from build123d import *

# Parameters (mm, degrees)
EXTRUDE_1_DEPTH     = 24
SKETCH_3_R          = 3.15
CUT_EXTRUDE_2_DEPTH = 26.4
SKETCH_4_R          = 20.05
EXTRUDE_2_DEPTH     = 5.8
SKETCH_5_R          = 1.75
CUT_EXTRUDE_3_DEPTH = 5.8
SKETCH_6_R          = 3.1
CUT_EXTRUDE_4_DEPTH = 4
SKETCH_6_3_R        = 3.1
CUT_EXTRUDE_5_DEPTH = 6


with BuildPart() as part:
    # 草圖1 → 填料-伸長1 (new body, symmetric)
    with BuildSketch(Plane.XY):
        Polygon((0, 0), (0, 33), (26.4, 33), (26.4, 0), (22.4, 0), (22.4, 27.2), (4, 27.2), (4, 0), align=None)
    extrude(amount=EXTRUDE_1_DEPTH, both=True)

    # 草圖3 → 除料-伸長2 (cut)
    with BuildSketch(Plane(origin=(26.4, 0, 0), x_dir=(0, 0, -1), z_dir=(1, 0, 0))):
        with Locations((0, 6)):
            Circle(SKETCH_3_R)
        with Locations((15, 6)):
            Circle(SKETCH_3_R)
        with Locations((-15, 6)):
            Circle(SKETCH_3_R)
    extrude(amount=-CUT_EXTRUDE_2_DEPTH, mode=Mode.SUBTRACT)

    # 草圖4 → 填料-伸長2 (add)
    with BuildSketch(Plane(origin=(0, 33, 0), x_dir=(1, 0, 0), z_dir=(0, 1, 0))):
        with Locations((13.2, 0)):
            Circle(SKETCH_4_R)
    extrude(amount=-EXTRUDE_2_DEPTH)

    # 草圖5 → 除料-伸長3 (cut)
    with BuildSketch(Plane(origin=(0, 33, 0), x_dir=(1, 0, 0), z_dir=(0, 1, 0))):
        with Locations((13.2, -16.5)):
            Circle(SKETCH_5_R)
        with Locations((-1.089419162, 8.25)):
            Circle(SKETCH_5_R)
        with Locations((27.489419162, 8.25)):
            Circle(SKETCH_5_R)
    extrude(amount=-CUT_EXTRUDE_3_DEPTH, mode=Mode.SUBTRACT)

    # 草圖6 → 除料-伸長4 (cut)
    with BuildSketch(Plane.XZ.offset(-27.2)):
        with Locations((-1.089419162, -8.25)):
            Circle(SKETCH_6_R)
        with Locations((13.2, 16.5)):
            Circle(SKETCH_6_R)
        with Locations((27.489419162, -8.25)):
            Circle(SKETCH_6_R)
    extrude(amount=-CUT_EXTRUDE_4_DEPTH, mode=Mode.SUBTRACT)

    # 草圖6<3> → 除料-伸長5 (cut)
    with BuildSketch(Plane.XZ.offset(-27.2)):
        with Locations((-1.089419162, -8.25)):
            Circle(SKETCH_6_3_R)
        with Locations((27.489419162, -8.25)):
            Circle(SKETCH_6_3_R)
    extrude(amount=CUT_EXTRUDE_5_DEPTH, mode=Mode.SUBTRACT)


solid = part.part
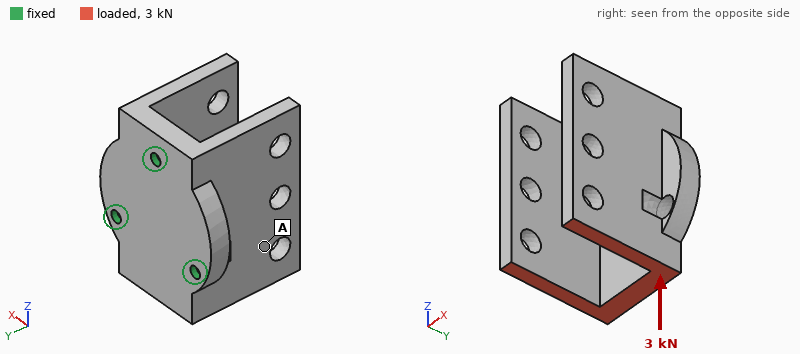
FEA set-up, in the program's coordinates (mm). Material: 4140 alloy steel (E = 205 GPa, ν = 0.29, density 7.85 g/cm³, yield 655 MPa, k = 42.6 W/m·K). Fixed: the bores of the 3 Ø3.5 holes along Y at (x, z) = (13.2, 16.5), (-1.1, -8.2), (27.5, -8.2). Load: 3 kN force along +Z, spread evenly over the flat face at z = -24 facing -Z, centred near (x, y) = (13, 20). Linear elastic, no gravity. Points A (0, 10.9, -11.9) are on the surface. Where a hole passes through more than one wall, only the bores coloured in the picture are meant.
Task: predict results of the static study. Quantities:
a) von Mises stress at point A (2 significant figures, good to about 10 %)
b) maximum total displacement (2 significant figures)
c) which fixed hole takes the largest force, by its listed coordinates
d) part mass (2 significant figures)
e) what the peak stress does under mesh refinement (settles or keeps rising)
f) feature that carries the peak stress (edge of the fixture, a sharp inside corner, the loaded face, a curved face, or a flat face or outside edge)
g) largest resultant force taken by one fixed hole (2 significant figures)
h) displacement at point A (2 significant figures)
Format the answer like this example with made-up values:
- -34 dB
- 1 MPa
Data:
- 15 MPa
- 21 µm
- (13.2, 16.5)
- 140 g
- keeps rising
- edge of the fixture
- 1.7 kN
- 12 µm
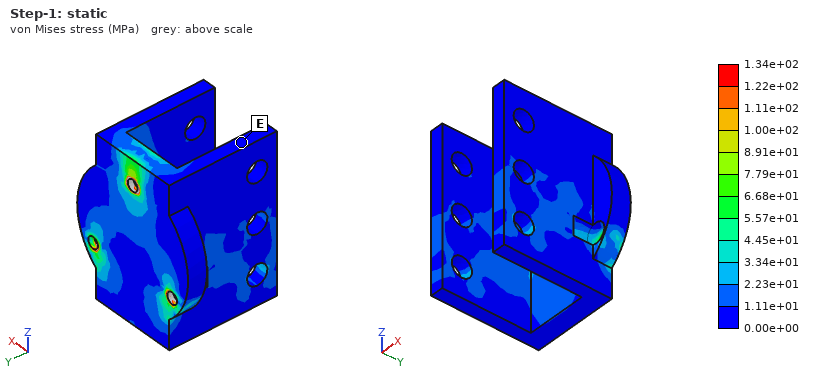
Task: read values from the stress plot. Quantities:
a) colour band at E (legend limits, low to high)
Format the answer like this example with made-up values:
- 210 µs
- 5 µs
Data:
- 0.00e+00 to 1.11e+01 MPa
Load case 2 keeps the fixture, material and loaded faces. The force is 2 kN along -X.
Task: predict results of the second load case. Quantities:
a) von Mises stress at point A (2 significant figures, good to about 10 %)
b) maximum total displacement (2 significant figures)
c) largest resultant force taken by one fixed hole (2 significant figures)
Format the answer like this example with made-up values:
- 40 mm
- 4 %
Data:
- 49 MPa
- 100 µm
- 1.7 kN
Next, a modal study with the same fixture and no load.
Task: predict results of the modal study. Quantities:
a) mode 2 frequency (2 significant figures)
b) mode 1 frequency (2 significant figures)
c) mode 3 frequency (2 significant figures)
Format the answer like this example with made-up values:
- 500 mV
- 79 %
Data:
- 3600 Hz
- 3500 Hz
- 5600 Hz
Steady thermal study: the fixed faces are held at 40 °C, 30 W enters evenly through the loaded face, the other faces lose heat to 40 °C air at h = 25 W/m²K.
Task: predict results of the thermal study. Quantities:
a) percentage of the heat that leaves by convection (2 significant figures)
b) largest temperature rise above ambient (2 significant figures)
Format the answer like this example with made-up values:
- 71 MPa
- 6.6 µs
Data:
- 23 %
- 70 K
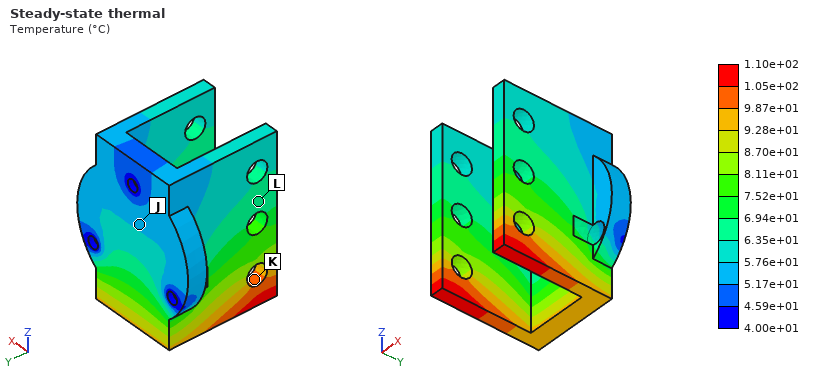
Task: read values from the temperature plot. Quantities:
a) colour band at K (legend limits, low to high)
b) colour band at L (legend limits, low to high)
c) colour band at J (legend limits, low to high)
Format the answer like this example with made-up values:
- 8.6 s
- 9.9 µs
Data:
- 9.87e+01 to 1.05e+02 °C
- 6.35e+01 to 6.94e+01 °C
- 5.17e+01 to 5.76e+01 °C
